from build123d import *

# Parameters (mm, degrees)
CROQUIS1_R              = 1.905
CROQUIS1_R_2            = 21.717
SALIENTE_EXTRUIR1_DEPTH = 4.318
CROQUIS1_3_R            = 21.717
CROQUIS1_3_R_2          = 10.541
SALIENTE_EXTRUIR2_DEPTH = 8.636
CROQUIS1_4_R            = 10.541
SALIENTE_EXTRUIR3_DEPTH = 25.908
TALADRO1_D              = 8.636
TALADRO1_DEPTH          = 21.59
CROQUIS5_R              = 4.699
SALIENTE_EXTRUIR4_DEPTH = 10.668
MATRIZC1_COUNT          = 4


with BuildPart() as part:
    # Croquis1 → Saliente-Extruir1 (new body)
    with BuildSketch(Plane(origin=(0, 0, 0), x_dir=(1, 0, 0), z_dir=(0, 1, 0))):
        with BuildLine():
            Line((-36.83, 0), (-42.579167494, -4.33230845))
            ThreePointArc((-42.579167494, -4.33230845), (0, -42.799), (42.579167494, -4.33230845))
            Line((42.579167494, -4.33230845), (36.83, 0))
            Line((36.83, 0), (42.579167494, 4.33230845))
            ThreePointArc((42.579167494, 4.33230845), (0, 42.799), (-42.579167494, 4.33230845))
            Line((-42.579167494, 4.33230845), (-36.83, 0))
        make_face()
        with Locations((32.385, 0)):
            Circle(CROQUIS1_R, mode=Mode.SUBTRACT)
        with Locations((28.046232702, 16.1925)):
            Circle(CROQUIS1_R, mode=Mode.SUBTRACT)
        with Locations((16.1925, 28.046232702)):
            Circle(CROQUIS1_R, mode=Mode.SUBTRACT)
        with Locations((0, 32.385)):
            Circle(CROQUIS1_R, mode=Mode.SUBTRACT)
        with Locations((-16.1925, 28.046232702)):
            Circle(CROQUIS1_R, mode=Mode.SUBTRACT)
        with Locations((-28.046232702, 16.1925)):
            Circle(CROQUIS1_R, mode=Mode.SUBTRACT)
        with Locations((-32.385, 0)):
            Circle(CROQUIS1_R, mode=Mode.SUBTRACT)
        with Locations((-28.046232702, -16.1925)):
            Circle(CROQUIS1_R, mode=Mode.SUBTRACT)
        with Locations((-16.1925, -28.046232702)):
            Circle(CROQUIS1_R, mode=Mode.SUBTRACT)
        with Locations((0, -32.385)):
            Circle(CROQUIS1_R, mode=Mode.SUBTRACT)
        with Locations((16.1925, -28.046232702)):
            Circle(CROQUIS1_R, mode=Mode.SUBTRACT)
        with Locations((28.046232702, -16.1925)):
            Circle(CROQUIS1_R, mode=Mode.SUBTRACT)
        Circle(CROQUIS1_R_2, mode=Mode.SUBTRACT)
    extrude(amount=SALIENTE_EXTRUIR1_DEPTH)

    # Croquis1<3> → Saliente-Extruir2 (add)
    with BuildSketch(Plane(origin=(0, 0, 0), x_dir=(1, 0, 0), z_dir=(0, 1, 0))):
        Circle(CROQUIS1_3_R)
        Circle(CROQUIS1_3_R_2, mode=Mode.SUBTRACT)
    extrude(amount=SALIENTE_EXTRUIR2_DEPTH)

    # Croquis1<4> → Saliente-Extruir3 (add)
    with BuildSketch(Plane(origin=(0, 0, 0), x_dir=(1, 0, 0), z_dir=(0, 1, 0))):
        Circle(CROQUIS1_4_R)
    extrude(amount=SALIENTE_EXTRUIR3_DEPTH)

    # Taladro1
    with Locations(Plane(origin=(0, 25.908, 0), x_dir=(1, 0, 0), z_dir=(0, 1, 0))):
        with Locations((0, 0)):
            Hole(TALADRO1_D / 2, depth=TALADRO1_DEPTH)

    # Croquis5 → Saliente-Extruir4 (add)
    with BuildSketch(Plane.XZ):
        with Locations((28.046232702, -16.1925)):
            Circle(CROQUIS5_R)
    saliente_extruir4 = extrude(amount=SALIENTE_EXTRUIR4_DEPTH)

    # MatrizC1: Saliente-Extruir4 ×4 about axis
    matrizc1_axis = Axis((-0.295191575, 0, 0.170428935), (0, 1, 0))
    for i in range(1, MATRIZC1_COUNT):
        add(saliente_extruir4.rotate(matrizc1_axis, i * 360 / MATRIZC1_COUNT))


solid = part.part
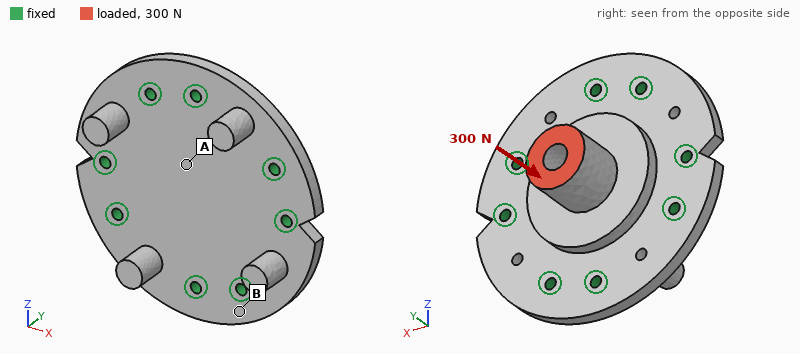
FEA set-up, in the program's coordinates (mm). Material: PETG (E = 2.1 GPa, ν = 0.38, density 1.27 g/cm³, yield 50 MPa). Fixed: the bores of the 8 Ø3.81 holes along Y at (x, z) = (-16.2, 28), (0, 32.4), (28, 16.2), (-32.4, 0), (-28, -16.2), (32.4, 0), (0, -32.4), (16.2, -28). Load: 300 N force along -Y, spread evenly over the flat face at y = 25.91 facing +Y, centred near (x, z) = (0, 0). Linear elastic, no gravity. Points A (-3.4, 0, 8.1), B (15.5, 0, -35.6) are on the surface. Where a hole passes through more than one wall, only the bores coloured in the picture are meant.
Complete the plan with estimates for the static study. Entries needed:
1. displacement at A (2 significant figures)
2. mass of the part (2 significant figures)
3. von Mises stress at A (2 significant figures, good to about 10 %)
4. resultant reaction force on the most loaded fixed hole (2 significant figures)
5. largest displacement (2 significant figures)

68 µm
48 g
1.9 MPa
52 N
77 µm
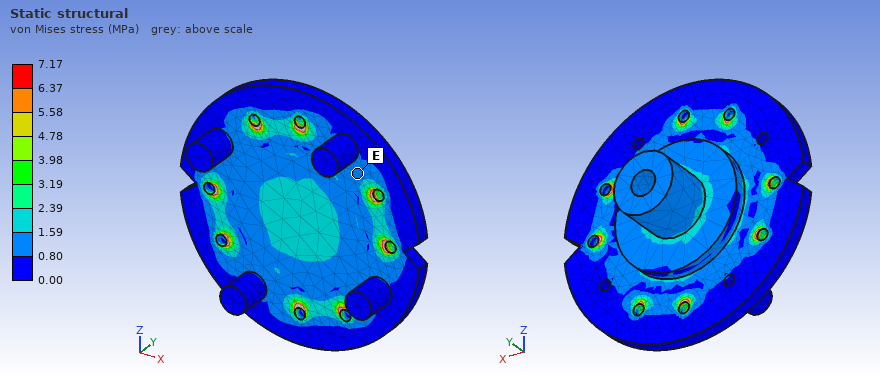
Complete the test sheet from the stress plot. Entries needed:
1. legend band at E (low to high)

0.80 to 1.59 MPa
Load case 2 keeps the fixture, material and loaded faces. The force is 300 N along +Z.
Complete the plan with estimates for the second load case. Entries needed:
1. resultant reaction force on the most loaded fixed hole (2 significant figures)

95 N
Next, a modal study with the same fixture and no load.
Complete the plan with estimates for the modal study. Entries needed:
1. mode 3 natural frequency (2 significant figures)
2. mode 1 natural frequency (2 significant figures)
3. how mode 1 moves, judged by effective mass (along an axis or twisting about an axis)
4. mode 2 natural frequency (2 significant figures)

2900 Hz
2300 Hz
along Y
2800 Hz
